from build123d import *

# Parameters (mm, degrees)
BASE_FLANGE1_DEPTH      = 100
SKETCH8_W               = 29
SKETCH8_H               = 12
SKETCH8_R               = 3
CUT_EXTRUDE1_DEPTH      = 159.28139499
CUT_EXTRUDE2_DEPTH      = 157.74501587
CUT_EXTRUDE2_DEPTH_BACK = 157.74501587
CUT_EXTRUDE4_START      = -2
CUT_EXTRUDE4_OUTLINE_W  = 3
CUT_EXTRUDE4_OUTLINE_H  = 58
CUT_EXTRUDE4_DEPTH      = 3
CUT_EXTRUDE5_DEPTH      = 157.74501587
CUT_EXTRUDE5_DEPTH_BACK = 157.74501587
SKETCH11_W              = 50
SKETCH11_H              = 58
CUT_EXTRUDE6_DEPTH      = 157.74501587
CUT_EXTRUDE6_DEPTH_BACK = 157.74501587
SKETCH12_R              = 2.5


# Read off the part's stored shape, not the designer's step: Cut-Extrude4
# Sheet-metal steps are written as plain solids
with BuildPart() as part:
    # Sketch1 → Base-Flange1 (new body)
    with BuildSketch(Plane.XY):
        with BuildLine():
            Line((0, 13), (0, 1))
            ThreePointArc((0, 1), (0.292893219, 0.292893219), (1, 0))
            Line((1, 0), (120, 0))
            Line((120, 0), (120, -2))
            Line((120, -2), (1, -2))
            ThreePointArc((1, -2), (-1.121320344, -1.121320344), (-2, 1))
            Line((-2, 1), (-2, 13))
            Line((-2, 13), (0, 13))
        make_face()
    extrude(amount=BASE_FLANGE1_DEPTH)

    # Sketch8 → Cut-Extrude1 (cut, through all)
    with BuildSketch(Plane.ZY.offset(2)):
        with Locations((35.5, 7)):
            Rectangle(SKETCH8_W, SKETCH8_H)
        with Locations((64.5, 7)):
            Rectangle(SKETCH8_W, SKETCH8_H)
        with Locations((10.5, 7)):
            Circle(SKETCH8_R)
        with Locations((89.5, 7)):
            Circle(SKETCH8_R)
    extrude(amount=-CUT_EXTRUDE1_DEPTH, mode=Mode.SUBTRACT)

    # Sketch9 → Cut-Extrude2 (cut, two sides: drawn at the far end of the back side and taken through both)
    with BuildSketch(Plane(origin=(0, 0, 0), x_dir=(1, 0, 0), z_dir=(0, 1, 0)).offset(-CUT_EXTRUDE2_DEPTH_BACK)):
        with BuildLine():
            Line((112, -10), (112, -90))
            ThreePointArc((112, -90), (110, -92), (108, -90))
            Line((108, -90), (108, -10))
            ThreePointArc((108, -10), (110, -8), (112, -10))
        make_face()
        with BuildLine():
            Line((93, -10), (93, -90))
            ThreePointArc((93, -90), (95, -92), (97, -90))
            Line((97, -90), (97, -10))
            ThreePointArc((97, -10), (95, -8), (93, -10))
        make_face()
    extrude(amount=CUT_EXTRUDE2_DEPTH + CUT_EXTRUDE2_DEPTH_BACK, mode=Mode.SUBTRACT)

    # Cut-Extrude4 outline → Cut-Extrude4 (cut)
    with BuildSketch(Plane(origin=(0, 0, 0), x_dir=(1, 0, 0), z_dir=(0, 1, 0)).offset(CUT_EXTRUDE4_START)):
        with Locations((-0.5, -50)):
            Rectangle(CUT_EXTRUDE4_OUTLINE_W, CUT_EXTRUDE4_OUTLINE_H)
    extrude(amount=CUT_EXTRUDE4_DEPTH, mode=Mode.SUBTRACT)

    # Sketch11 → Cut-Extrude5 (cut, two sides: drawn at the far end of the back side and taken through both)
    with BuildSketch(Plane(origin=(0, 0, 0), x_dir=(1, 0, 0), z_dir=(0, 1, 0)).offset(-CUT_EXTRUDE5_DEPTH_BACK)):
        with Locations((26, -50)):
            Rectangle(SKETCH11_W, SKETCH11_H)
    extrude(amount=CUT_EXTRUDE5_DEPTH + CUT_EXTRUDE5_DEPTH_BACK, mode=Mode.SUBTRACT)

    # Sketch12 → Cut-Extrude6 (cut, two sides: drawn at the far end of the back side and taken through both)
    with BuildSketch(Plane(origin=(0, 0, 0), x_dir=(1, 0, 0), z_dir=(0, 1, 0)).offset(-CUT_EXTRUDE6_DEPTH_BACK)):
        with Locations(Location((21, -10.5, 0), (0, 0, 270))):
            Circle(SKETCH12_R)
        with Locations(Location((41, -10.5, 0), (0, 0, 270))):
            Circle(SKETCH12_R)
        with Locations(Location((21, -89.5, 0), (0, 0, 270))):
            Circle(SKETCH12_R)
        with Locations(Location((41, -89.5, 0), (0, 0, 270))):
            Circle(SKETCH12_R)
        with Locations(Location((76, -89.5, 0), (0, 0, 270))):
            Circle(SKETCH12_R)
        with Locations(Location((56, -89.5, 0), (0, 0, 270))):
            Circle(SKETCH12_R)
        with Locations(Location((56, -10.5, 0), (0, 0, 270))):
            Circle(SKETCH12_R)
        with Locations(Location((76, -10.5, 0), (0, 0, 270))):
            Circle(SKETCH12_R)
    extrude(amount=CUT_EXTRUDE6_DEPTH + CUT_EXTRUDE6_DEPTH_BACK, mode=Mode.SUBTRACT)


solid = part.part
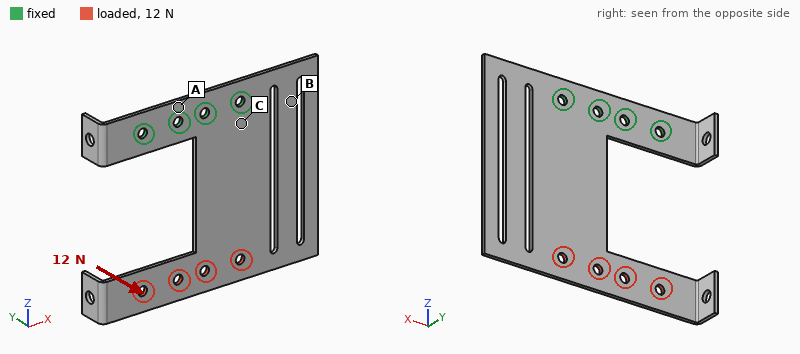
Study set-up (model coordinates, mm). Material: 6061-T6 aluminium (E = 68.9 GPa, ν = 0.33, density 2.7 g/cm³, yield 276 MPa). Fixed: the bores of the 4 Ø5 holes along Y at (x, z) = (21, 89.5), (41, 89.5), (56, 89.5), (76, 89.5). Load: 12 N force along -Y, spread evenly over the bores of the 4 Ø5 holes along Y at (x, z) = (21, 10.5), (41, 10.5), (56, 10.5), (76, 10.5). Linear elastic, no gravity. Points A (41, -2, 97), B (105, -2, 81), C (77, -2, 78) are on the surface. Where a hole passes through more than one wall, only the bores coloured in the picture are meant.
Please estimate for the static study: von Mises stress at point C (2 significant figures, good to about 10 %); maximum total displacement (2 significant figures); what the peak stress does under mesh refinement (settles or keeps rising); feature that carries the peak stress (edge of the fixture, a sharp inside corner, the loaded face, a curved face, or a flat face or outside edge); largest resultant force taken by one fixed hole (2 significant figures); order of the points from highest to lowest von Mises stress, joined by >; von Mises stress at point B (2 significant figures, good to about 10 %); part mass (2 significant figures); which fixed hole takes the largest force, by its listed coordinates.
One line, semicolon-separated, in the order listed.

22 MPa; 1.6 mm; keeps rising; edge of the fixture; 13 N; C > B > A; 8.9 MPa; 47 g; (56, 89.5)
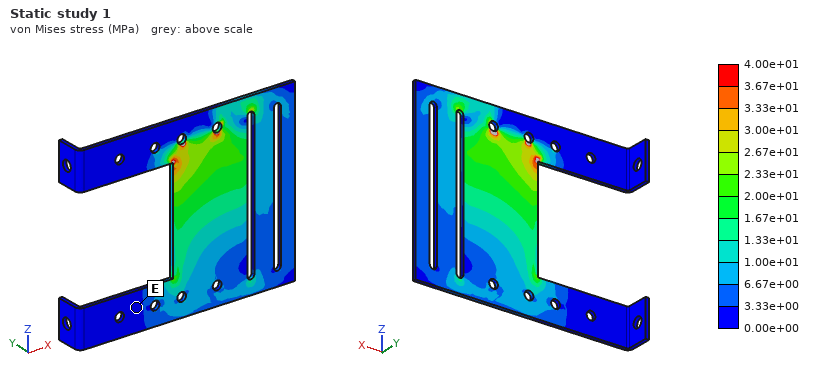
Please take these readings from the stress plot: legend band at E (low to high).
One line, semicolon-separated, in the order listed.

0.00e+00 to 3.33e+00 MPa
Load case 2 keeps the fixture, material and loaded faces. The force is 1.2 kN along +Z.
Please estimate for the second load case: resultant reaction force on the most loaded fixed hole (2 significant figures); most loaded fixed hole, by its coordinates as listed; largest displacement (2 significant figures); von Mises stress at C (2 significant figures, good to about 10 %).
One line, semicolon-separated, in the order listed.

1.1 kN; (56, 89.5); 0.38 mm; 12 MPa
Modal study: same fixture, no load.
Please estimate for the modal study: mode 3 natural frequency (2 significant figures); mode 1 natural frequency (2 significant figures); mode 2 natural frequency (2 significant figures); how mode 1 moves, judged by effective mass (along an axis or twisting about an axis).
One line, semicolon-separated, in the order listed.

510 Hz; 130 Hz; 210 Hz; along Y
